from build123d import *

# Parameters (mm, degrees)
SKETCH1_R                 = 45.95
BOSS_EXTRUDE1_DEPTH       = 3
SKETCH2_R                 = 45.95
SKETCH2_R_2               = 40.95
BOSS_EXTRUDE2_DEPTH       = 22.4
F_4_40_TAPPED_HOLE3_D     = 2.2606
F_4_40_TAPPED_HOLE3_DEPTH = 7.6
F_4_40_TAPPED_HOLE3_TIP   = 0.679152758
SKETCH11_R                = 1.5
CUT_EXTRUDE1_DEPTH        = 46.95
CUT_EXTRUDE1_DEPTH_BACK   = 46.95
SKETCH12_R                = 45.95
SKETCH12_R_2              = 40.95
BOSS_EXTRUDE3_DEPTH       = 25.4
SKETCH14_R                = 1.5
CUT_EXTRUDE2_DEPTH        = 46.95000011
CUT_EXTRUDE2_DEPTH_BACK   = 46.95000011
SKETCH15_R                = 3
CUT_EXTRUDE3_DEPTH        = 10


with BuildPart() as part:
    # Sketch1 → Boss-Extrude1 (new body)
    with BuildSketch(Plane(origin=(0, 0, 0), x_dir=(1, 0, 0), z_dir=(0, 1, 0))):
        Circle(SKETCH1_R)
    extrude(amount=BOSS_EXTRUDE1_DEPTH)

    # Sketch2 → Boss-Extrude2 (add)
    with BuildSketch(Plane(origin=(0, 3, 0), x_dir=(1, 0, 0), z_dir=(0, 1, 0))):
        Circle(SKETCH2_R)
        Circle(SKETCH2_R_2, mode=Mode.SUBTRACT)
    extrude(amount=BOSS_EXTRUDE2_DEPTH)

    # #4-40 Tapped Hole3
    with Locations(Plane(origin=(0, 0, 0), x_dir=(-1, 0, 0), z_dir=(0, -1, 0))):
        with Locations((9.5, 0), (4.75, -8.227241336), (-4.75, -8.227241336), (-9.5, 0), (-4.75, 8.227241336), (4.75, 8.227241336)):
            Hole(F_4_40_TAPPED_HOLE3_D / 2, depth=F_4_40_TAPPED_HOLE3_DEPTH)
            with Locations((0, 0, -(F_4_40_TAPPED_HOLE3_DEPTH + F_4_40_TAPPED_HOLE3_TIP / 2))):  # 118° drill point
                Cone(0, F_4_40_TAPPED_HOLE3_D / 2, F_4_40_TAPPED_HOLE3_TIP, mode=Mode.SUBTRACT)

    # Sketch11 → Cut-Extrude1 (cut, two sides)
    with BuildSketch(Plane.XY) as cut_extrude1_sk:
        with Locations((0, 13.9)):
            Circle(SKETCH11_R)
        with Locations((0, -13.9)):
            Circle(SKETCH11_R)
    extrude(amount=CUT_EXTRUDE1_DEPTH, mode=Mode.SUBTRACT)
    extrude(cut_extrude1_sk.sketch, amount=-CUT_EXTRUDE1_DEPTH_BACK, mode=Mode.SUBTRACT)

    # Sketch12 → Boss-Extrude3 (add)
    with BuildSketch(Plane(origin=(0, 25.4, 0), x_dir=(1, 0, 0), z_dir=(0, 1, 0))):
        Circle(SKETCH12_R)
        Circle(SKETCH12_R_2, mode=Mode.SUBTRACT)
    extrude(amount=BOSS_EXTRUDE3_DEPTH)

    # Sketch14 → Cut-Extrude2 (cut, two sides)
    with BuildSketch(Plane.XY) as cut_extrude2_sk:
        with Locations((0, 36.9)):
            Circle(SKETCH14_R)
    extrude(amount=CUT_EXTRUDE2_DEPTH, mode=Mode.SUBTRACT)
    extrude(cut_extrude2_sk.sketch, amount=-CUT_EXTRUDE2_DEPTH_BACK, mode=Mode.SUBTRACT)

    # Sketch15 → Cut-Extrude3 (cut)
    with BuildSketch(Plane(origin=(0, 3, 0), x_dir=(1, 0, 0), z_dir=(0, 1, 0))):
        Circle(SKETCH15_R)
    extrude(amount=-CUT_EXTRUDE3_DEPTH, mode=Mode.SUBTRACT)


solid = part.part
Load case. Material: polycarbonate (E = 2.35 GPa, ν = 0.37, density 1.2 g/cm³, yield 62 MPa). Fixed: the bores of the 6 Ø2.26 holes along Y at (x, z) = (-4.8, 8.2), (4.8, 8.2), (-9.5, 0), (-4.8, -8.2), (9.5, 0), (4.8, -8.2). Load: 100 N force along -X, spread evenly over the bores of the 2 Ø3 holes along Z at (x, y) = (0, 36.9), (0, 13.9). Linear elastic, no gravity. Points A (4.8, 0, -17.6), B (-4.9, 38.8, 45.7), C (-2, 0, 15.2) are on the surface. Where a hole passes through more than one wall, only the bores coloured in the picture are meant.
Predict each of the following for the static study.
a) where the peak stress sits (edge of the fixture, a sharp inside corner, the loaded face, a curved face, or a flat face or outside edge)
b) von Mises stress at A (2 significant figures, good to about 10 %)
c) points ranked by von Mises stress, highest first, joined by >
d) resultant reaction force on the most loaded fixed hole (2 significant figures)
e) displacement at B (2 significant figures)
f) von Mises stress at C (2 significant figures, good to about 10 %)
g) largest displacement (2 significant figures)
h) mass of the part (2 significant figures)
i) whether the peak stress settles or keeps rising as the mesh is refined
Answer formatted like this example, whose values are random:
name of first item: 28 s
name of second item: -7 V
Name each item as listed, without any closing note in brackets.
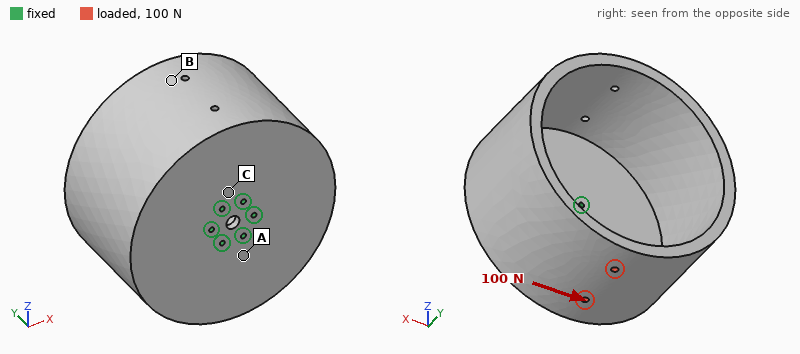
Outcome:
where the peak stress sits: edge of the fixture
von Mises stress at A: 3.2 MPa
points ranked by von Mises stress, highest first, joined by >: C > A > B
resultant reaction force on the most loaded fixed hole: 96 N
displacement at B: 0.71 mm
von Mises stress at C: 6.1 MPa
largest displacement: 1.4 mm
mass of the part: 100 g
whether the peak stress settles or keeps rising as the mesh is refined: keeps rising
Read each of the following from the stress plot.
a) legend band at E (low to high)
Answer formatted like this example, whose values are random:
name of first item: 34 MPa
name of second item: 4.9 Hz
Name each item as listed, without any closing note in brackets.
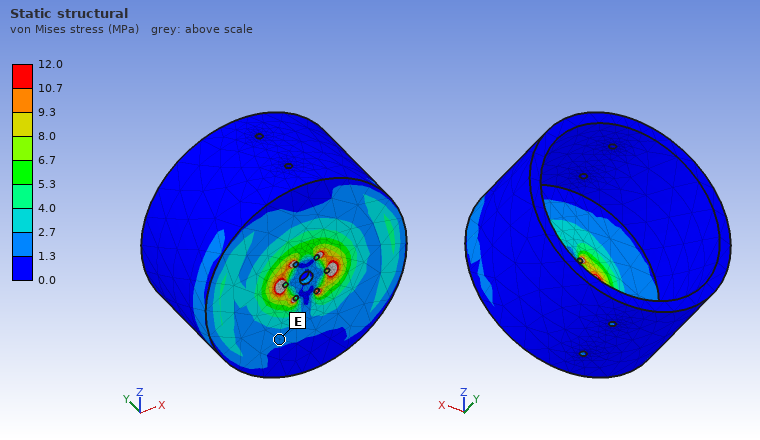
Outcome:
legend band at E: 1.3 to 2.7 MPa
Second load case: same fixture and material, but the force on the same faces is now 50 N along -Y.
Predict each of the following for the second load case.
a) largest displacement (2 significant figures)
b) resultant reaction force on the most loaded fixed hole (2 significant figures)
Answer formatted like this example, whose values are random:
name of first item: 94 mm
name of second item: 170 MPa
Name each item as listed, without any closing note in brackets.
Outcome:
largest displacement: 1.4 mm
resultant reaction force on the most loaded fixed hole: 46 N
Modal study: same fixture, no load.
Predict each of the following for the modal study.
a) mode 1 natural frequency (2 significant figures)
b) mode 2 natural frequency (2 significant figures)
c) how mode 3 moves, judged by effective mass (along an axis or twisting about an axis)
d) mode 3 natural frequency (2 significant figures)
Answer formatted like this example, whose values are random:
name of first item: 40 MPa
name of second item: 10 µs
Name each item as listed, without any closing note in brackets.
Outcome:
mode 1 natural frequency: 140 Hz
mode 2 natural frequency: 140 Hz
how mode 3 moves, judged by effective mass: along Y
mode 3 natural frequency: 300 Hz
